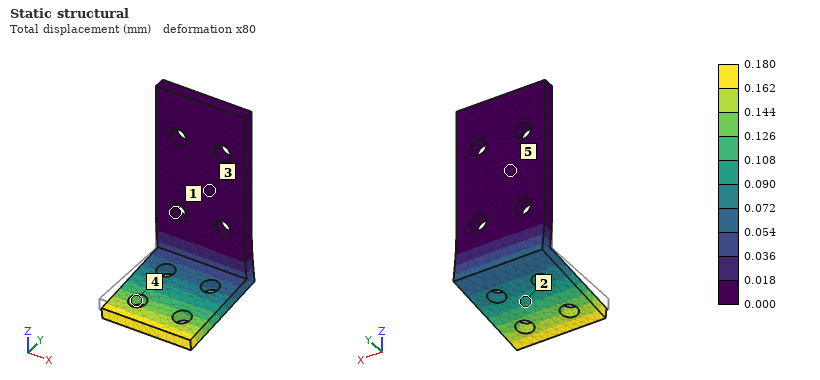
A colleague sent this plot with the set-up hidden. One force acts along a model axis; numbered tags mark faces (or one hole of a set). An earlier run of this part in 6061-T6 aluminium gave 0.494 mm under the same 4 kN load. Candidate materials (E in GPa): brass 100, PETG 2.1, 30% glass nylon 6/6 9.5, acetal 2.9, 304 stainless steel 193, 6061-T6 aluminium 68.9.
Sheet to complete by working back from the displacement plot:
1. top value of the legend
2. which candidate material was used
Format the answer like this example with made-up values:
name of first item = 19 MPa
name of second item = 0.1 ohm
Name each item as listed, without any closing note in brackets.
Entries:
top value of the legend = 0.180 mm
which candidate material was used = 304 stainless steel
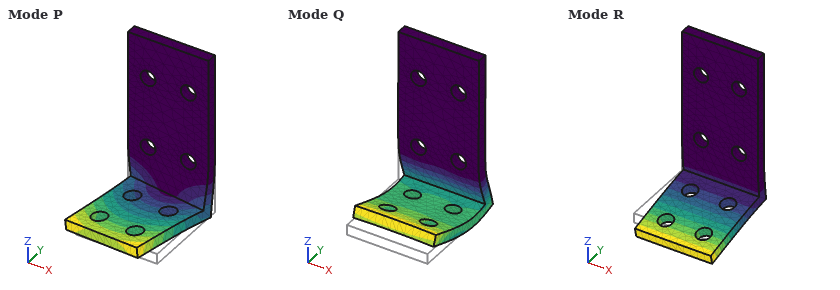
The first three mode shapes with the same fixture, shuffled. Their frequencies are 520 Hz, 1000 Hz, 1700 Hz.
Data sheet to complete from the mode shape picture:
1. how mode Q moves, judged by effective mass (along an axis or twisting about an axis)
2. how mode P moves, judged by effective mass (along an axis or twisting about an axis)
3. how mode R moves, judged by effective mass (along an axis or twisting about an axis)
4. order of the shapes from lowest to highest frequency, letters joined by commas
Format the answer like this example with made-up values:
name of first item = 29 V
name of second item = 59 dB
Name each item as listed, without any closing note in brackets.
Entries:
how mode Q moves, judged by effective mass = along Y
how mode P moves, judged by effective mass = along X
how mode R moves, judged by effective mass = along Z
order of the shapes from lowest to highest frequency, letters joined by commas = R, P, Q
